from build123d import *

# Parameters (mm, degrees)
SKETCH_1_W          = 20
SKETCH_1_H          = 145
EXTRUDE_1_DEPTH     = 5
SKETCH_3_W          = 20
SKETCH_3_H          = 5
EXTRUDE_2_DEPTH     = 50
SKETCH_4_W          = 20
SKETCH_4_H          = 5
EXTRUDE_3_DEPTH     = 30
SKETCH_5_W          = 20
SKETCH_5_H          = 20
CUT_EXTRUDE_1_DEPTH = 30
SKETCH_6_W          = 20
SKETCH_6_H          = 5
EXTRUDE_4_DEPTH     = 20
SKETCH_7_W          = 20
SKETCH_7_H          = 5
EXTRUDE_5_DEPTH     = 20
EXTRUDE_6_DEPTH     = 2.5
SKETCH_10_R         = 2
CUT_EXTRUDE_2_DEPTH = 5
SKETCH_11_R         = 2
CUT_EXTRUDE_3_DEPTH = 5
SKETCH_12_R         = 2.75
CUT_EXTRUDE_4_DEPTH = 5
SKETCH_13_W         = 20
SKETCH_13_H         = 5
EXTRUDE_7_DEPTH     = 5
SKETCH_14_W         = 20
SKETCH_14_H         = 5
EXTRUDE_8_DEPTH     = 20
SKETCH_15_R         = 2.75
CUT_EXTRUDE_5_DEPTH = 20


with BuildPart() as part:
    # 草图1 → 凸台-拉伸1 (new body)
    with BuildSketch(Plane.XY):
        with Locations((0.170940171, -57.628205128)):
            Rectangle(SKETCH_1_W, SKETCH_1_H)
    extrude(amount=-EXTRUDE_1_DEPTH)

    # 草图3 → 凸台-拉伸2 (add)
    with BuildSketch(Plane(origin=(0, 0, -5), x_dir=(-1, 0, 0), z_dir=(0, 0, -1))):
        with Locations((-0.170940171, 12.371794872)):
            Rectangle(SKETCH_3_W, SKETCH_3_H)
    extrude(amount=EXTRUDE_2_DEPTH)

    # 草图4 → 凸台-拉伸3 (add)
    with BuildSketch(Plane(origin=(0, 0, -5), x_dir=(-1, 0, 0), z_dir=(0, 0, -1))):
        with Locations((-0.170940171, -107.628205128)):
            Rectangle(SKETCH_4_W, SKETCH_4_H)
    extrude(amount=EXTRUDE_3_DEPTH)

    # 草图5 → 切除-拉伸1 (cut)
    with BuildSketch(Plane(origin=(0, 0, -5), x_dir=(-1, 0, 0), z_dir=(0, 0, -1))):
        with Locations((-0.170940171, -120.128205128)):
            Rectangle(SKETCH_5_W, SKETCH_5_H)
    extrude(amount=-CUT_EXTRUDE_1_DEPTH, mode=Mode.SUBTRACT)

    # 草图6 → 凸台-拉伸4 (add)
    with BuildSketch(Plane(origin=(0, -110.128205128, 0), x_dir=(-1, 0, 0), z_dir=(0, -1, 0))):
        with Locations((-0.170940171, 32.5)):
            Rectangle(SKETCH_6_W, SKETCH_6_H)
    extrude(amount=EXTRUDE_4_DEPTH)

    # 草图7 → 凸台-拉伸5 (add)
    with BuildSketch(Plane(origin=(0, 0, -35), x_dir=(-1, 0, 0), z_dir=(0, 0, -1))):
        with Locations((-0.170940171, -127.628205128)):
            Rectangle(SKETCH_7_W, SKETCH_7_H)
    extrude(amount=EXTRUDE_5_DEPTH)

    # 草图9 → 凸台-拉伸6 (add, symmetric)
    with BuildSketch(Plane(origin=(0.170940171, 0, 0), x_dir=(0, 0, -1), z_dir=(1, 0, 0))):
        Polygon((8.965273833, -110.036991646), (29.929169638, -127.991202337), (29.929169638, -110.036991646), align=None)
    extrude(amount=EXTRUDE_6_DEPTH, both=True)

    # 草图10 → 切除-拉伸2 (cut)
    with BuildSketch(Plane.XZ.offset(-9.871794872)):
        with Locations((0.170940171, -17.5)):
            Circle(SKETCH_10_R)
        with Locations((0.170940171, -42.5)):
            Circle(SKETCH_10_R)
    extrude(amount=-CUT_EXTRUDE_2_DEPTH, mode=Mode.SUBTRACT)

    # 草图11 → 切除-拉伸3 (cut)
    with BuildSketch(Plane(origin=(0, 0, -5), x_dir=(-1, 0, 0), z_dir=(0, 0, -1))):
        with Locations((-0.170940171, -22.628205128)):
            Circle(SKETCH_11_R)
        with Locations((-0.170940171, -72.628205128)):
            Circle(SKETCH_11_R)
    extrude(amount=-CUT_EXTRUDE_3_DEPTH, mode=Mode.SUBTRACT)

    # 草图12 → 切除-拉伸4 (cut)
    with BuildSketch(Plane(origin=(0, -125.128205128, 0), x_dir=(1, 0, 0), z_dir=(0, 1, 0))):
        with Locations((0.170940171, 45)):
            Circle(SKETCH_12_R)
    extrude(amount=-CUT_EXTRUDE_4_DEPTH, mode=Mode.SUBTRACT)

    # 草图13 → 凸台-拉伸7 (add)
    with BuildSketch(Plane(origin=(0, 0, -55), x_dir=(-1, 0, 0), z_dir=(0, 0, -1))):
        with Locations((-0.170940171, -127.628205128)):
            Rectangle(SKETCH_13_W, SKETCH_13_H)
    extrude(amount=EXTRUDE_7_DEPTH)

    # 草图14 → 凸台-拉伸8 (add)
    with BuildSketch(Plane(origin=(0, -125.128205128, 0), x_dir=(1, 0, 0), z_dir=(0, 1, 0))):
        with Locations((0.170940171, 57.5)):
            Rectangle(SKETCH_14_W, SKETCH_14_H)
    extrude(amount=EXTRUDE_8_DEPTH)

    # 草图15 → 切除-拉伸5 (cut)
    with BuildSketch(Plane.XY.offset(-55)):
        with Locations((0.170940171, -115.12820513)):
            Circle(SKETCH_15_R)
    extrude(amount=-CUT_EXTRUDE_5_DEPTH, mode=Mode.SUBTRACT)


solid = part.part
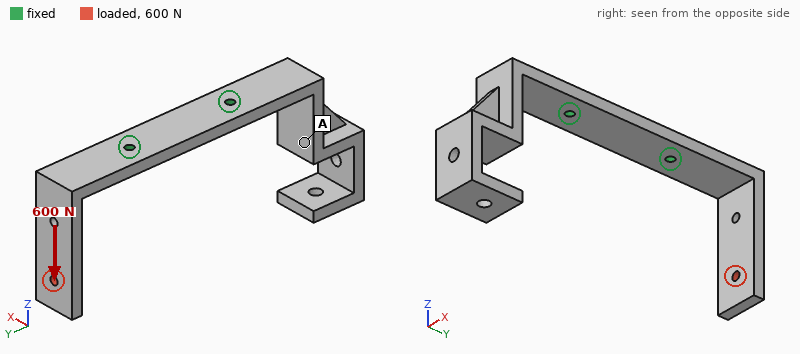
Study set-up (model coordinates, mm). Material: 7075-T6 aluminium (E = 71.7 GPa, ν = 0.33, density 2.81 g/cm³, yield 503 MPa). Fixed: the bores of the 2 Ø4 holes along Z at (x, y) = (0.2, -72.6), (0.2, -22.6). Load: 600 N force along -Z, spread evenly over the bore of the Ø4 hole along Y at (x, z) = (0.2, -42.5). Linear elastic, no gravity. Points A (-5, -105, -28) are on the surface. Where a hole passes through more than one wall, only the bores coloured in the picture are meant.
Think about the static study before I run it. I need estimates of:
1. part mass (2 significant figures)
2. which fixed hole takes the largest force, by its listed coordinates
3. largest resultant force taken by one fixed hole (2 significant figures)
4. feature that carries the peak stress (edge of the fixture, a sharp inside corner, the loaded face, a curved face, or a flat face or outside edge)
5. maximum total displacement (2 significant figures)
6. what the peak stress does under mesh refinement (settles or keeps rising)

77 g
(0.2, -22.6)
650 N
edge of the fixture
1.4 mm
keeps rising
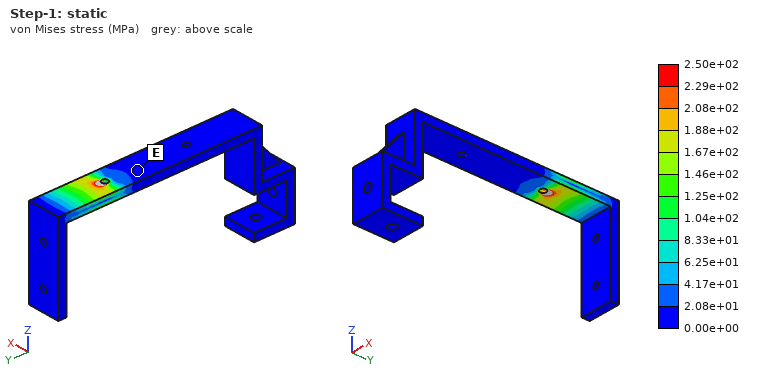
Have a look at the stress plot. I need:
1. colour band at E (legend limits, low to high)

0.00e+00 to 2.08e+01 MPa
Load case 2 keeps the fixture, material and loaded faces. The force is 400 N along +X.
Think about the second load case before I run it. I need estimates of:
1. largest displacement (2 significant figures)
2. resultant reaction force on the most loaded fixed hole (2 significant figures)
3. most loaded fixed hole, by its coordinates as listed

1.5 mm
600 N
(0.2, -22.6)
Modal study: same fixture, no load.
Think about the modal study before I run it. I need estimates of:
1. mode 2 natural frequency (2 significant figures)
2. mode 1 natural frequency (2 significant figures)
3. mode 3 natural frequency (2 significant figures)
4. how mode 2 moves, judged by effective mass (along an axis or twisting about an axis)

580 Hz
380 Hz
700 Hz
along X
